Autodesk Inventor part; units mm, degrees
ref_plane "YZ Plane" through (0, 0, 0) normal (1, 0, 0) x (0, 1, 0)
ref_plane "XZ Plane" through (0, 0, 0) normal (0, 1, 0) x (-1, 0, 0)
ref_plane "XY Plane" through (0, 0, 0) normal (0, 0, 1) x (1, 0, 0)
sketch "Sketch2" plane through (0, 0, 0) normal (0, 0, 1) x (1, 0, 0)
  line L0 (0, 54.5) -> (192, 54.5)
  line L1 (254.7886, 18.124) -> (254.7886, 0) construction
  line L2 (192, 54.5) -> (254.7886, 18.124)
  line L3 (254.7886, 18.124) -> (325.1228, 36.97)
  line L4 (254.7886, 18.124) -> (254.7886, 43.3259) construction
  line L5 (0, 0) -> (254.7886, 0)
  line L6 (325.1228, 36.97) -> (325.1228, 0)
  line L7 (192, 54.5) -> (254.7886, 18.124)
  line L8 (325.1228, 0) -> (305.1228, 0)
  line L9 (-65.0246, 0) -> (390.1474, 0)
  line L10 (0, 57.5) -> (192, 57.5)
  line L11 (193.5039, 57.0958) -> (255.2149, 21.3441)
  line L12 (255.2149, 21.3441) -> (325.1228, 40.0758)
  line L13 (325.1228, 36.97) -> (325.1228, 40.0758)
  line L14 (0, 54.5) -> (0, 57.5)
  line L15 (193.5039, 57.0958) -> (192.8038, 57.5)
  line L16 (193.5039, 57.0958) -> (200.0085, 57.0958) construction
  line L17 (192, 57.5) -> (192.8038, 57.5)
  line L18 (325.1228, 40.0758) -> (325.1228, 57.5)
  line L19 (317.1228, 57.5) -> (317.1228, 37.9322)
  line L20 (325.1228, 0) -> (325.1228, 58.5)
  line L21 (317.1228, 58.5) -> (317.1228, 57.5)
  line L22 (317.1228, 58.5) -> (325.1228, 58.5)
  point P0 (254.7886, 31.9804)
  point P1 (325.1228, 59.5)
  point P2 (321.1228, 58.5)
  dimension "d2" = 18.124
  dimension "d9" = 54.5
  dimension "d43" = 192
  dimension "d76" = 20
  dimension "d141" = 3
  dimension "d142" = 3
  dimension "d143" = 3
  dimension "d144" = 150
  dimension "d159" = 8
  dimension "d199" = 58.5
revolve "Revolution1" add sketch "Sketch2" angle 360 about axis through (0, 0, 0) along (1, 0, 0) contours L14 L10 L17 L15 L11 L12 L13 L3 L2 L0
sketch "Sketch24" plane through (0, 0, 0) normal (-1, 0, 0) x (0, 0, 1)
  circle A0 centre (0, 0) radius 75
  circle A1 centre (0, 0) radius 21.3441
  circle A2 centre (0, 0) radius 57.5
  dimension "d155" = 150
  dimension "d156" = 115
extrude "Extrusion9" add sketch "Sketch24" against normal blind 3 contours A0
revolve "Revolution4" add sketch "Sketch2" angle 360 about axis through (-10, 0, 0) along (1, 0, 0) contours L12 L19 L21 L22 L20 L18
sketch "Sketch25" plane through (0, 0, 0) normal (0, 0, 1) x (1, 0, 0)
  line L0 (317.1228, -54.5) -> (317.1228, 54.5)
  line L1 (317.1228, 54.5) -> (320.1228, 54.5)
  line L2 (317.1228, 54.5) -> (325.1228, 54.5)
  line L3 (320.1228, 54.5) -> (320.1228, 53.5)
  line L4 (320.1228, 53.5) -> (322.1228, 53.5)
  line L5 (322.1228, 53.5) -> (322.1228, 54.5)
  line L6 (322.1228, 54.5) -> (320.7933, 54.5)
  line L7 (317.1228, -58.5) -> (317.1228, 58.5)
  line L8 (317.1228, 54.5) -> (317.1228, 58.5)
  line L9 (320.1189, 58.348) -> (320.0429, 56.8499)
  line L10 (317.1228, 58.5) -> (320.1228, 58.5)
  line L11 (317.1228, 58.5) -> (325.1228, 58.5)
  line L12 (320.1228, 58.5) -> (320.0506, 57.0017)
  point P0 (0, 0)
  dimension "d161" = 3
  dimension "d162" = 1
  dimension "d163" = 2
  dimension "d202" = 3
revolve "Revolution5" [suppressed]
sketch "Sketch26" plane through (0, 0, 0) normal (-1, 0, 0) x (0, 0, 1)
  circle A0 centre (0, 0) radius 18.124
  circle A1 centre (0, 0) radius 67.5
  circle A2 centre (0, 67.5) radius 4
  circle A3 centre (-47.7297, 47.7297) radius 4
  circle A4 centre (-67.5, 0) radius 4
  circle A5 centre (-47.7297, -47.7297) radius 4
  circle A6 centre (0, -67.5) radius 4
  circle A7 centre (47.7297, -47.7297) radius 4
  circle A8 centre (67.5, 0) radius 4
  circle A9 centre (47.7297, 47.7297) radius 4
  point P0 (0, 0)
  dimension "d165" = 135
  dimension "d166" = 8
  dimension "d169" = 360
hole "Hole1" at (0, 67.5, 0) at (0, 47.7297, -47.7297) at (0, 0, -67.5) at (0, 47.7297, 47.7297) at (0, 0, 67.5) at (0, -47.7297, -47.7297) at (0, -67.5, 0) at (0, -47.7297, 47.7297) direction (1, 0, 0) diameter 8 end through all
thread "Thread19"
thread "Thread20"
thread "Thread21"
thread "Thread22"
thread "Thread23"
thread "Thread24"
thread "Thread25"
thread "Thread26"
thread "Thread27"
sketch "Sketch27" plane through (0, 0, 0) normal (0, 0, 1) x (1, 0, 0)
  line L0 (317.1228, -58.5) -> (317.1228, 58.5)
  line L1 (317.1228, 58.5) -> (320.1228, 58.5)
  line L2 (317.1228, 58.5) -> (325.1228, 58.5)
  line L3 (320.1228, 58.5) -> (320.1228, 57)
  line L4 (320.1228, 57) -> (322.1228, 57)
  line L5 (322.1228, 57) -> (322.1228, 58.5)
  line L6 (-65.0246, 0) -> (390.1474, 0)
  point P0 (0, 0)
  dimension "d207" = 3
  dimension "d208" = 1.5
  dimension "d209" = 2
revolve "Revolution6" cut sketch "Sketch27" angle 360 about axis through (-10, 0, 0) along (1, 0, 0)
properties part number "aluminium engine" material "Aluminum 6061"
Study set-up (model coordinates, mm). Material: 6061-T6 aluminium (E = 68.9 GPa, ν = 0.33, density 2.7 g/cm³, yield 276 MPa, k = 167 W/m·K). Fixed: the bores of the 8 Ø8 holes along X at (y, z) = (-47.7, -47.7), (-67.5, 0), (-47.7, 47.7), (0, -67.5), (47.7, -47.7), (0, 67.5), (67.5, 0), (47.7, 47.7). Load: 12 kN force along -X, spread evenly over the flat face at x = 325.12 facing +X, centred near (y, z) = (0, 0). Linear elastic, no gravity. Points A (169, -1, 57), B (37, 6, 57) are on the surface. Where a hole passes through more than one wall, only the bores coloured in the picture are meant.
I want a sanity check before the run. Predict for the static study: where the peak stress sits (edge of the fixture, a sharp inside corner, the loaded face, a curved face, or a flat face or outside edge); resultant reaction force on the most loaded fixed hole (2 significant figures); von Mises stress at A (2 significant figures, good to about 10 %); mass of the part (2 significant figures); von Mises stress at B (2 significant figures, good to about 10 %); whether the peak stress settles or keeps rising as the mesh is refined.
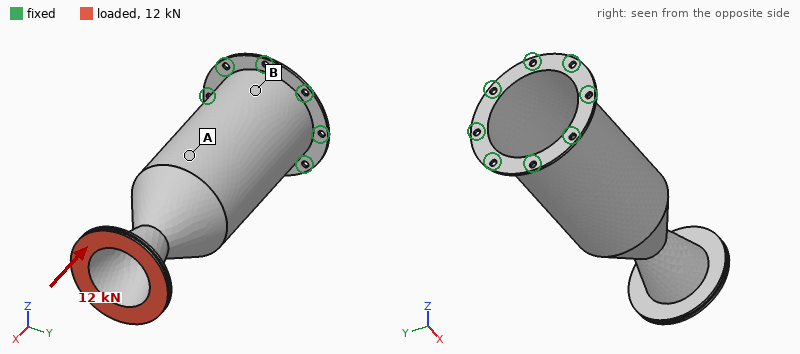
edge of the fixture
1.6 kN
15 MPa
980 g
9.0 MPa
keeps rising
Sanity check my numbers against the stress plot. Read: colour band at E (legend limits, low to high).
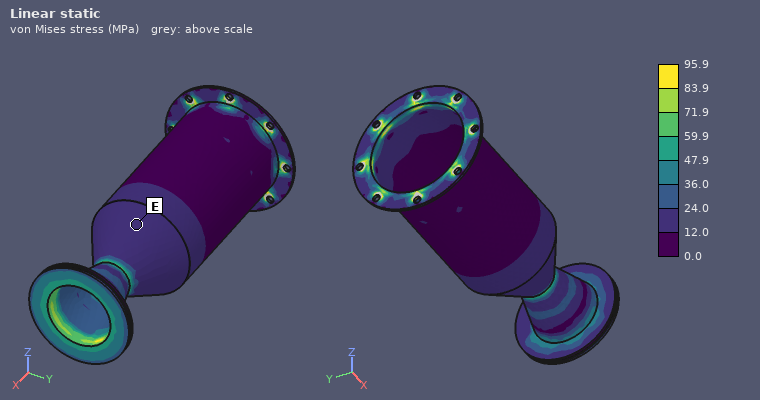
12.0 to 24.0 MPa
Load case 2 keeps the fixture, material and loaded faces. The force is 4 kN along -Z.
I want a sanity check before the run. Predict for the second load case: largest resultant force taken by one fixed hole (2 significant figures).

5.7 kN
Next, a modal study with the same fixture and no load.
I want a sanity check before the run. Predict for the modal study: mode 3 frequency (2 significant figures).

1800 Hz
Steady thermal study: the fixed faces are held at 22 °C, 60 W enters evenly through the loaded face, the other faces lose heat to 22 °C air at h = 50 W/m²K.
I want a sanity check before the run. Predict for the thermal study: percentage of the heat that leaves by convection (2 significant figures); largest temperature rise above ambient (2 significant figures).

99 %
32 K
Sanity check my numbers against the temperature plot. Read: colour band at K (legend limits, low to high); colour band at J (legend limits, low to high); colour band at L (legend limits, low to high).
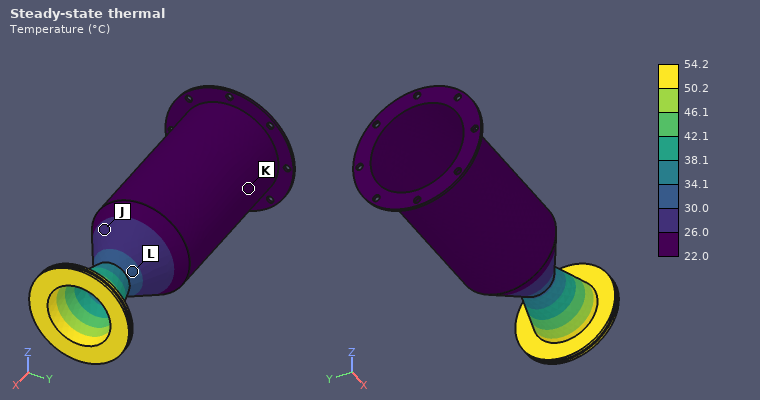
22.0 to 26.0 °C
26.0 to 30.0 °C
30.0 to 34.1 °C
